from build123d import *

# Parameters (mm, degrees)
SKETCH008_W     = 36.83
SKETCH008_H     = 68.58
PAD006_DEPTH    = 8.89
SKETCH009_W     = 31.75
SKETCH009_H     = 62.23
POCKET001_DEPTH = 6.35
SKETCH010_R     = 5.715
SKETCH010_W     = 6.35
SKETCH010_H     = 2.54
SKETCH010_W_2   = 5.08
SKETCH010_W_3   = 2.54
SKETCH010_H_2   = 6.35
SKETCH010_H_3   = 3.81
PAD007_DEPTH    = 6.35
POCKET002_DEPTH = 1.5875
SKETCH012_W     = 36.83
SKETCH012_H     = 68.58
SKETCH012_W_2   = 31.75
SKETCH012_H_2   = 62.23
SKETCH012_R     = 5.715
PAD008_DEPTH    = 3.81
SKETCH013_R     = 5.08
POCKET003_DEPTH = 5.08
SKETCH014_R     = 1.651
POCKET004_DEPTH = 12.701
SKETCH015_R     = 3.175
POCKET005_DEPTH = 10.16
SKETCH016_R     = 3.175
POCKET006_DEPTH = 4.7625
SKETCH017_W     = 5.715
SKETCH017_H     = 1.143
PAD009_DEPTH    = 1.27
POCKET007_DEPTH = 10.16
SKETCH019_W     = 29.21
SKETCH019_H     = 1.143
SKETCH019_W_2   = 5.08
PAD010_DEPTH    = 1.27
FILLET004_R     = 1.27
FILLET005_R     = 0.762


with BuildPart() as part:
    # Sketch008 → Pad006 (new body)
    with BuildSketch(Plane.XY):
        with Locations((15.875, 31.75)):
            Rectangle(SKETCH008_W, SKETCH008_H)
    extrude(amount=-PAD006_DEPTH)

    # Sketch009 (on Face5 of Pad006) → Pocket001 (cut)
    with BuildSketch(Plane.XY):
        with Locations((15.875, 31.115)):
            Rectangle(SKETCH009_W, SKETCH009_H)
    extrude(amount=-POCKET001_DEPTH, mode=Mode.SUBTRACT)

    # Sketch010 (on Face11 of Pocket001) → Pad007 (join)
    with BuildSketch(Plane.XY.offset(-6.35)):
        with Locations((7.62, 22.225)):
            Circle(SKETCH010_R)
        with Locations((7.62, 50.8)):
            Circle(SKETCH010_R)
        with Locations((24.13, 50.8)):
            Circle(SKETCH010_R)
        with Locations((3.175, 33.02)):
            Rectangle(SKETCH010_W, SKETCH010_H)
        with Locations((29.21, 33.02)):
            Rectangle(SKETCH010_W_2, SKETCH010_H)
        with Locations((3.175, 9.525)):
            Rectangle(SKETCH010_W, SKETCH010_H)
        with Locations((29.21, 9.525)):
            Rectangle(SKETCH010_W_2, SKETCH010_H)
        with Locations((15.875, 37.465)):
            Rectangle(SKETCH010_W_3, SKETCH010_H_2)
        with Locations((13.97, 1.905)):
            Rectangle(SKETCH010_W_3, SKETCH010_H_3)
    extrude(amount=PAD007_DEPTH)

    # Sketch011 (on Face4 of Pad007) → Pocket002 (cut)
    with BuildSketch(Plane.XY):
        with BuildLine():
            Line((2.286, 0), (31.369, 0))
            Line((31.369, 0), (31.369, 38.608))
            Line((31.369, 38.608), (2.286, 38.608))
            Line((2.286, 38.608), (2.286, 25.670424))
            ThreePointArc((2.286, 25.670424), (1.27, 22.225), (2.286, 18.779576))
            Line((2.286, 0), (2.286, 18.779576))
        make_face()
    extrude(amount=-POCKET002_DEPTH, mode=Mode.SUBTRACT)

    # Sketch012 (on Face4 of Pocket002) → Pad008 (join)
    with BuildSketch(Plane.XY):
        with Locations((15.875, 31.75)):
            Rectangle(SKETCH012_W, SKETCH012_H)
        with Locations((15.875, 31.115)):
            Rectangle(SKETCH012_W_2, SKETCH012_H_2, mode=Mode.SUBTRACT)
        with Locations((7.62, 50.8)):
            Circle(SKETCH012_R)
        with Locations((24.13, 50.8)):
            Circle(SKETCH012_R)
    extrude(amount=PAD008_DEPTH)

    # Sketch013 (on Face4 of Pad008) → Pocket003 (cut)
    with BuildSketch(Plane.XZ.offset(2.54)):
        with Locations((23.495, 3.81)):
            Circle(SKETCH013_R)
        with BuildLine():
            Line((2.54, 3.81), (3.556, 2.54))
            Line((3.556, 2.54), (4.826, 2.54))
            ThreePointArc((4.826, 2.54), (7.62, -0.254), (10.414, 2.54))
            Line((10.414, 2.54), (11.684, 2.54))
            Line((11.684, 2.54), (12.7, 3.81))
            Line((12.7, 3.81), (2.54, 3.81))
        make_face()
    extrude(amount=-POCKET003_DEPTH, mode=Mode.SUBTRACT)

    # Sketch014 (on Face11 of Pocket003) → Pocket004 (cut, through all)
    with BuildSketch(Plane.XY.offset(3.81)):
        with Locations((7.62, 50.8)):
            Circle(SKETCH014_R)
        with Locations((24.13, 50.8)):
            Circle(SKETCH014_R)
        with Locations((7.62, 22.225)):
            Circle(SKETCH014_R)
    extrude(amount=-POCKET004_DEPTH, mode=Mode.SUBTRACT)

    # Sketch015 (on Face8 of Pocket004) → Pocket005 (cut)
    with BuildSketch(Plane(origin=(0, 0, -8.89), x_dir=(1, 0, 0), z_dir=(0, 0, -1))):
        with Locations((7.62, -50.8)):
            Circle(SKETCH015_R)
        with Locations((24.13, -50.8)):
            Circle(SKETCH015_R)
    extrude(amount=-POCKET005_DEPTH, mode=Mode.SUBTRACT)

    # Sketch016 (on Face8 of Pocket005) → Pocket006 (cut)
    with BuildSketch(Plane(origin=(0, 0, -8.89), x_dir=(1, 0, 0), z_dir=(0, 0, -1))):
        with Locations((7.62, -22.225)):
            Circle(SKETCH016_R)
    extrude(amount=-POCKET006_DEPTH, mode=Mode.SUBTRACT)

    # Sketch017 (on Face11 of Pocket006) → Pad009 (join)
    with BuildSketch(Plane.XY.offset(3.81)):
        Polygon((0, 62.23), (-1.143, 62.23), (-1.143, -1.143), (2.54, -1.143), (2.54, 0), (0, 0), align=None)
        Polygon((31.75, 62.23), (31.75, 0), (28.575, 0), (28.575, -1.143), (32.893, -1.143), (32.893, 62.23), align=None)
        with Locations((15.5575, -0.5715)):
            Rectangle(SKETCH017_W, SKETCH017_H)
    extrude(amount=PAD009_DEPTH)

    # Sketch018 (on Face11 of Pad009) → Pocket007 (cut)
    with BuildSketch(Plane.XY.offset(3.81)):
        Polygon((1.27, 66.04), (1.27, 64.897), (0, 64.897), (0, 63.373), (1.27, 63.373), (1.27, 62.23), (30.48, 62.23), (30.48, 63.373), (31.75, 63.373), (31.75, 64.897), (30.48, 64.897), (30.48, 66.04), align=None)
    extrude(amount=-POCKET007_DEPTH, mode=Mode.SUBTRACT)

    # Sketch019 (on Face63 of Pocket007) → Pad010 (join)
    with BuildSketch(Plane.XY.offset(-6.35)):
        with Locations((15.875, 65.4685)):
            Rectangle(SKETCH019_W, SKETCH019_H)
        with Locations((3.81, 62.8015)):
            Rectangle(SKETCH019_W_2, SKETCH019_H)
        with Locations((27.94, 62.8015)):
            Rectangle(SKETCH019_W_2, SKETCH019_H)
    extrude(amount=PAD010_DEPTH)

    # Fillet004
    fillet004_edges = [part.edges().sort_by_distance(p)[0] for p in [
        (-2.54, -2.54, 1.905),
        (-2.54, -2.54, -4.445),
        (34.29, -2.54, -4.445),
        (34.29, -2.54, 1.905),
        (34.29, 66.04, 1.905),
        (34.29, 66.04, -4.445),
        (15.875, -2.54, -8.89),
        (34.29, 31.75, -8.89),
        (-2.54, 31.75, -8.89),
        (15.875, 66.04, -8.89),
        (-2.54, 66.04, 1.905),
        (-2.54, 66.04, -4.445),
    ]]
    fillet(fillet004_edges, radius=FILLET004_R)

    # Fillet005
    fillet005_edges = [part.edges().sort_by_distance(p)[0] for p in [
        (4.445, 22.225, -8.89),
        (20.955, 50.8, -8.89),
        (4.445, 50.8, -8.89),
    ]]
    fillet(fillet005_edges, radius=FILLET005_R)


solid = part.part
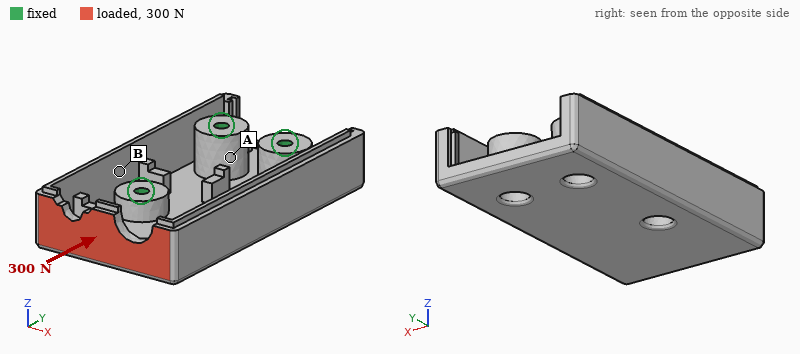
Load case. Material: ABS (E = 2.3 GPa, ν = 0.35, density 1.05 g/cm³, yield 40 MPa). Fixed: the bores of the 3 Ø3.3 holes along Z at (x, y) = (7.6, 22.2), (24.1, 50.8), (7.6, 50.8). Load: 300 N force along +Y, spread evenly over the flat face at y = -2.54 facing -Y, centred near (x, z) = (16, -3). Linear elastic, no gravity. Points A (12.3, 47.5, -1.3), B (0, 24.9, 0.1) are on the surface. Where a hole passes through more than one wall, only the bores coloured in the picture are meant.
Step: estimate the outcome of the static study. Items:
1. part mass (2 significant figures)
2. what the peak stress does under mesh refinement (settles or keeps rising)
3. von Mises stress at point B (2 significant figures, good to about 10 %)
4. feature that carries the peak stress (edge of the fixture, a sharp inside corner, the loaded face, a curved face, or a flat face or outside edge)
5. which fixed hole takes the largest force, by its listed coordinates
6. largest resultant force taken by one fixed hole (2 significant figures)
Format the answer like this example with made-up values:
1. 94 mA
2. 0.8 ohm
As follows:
1. 14 g
2. keeps rising
3. 3.6 MPa
4. edge of the fixture
5. (7.6, 22.2)
6. 190 N
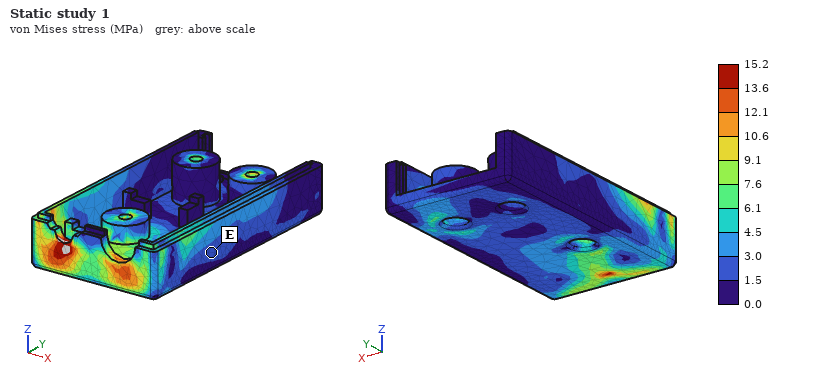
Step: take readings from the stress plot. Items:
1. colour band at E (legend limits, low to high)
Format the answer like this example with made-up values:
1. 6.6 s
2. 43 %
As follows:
1. 1.5 to 3.0 MPa
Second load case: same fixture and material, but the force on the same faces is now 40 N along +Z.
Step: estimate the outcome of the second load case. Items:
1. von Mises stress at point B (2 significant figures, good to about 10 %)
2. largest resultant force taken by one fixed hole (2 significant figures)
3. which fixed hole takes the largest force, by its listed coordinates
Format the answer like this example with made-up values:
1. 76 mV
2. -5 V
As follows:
1. 1.4 MPa
2. 62 N
3. (7.6, 22.2)
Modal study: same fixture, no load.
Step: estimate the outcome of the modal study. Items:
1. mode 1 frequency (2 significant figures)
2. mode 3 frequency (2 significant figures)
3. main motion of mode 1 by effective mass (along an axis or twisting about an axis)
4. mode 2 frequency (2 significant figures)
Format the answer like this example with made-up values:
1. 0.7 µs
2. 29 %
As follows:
1. 680 Hz
2. 1800 Hz
3. along Z
4. 1600 Hz
